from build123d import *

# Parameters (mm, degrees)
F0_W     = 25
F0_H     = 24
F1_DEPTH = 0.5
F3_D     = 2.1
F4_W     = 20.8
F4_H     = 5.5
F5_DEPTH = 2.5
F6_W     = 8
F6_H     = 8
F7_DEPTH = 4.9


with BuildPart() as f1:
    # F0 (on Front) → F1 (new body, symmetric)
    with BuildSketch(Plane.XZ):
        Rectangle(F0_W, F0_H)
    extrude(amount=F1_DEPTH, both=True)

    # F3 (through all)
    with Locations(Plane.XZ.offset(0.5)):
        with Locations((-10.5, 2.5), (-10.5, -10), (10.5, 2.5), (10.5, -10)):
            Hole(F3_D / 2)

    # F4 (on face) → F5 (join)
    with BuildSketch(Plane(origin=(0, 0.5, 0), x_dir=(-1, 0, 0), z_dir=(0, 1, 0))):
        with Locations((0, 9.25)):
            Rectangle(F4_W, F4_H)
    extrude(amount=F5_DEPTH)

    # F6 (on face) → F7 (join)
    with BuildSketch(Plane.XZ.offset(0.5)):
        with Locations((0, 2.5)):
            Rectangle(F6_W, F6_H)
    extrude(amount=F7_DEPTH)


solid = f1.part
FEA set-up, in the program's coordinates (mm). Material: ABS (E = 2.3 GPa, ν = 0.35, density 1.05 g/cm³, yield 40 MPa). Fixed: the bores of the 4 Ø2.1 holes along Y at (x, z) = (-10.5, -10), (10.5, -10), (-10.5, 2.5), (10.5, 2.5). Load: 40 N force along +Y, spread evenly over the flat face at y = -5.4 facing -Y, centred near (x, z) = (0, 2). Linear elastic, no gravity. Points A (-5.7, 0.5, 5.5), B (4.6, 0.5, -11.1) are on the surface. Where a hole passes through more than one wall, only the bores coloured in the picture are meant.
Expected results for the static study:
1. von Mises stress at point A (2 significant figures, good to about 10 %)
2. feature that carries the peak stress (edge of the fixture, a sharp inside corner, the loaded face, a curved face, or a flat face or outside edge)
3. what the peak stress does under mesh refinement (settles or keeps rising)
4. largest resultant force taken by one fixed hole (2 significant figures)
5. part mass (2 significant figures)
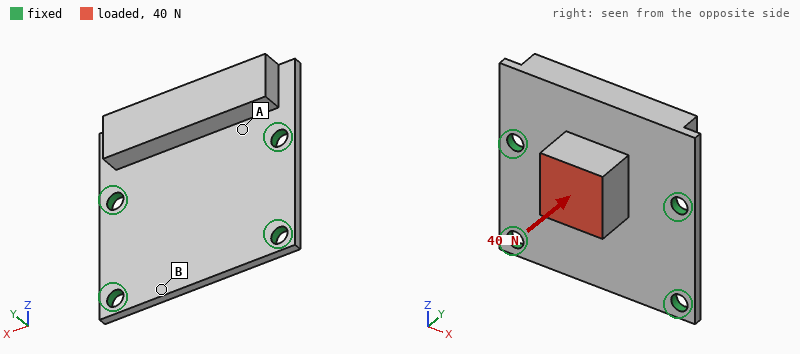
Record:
8.5 MPa
edge of the fixture
keeps rising
18 N
1.2 g
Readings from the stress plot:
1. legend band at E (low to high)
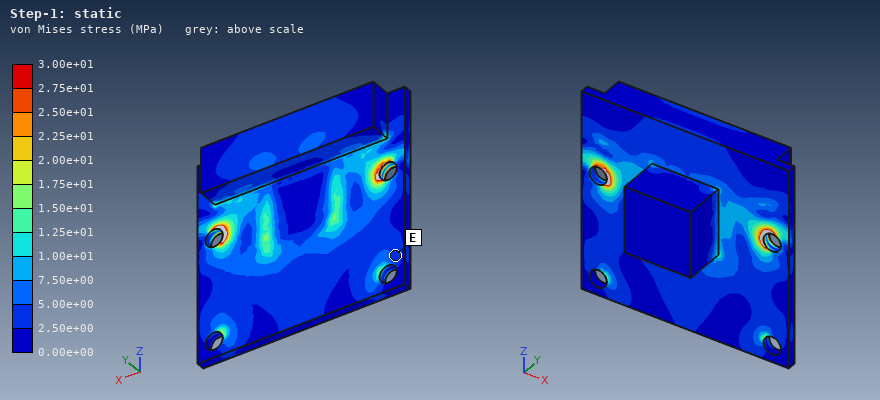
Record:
2.50e+00 to 5.00e+00 MPa
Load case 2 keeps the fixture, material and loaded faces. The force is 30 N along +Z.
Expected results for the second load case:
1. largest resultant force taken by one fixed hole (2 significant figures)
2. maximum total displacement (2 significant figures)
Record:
12 N
0.36 mm
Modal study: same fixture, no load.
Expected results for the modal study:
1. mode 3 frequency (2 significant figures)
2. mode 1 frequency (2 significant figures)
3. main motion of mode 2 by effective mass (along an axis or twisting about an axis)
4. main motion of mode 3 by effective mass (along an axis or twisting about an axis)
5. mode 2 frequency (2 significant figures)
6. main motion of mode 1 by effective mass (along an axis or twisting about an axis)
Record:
5000 Hz
1700 Hz
along Y
twisting about Z
3200 Hz
along Y
